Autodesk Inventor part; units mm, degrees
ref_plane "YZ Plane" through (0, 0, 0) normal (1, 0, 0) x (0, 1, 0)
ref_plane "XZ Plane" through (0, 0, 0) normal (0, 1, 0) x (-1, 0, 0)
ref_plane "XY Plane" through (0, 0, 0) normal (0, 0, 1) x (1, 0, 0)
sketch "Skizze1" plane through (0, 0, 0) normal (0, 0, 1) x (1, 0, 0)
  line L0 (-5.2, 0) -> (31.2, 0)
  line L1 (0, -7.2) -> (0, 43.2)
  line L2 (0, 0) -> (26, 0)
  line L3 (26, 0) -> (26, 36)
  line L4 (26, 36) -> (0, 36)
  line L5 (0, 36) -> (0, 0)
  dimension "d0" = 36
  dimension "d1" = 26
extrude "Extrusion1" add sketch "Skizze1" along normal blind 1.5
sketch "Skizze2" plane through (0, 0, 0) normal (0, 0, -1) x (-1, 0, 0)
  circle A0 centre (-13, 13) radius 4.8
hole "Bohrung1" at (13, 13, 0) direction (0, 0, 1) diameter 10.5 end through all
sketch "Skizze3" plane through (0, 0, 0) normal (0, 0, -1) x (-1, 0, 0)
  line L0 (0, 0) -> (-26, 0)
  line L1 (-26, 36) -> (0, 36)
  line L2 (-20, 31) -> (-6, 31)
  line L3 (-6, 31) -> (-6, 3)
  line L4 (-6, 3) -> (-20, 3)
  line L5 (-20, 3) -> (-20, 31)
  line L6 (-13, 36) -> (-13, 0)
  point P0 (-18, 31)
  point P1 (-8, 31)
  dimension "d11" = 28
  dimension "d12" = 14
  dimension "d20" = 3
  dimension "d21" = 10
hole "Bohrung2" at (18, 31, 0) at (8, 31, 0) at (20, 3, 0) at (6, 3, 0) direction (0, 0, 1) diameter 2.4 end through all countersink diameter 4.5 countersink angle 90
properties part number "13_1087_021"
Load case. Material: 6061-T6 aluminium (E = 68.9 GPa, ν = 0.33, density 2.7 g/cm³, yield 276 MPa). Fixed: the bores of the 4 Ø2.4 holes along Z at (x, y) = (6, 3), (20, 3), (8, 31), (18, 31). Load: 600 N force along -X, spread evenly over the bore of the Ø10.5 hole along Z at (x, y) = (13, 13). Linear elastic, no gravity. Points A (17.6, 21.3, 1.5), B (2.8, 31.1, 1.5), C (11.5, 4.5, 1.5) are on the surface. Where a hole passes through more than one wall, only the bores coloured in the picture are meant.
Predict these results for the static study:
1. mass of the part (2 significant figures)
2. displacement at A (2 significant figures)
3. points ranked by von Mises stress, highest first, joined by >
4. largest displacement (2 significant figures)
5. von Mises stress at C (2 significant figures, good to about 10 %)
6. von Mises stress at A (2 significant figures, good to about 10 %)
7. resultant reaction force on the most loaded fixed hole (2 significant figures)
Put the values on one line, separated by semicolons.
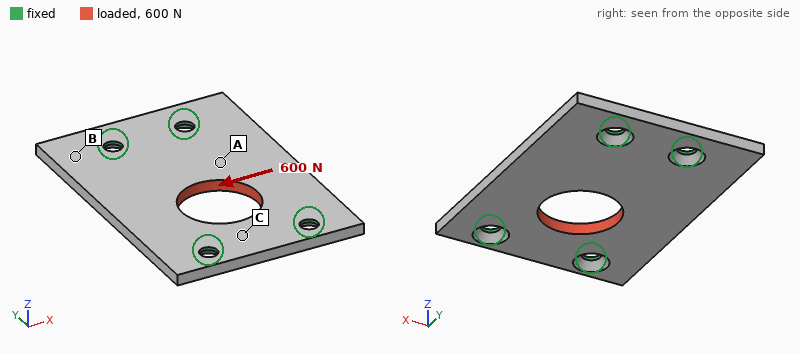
3.3 g; 4.6 µm; C > A > B; 6.8 µm; 23 MPa; 12 MPa; 180 N
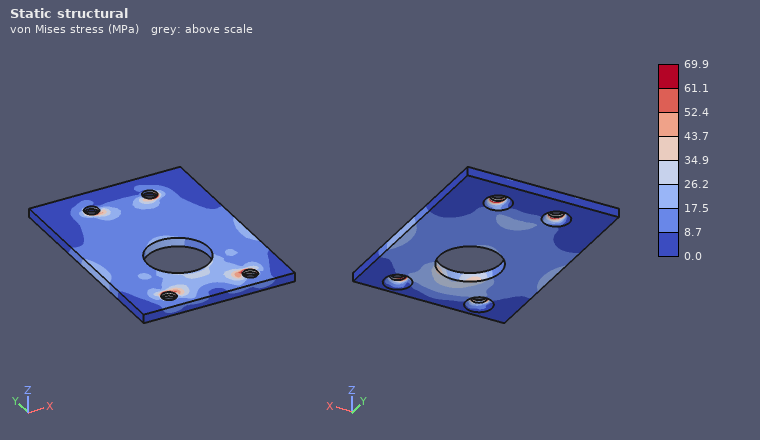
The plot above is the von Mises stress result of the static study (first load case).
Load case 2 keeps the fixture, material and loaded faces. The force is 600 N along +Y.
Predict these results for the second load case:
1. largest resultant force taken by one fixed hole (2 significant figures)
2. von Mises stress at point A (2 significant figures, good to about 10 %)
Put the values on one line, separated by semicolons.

180 N; 13 MPa
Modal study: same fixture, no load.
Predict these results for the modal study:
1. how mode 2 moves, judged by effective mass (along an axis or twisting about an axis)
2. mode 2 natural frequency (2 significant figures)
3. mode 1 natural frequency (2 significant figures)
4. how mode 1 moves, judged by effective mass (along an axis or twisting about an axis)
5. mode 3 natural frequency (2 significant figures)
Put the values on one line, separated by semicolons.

twisting about Y; 8500 Hz; 7600 Hz; along Z; 14 kHz
